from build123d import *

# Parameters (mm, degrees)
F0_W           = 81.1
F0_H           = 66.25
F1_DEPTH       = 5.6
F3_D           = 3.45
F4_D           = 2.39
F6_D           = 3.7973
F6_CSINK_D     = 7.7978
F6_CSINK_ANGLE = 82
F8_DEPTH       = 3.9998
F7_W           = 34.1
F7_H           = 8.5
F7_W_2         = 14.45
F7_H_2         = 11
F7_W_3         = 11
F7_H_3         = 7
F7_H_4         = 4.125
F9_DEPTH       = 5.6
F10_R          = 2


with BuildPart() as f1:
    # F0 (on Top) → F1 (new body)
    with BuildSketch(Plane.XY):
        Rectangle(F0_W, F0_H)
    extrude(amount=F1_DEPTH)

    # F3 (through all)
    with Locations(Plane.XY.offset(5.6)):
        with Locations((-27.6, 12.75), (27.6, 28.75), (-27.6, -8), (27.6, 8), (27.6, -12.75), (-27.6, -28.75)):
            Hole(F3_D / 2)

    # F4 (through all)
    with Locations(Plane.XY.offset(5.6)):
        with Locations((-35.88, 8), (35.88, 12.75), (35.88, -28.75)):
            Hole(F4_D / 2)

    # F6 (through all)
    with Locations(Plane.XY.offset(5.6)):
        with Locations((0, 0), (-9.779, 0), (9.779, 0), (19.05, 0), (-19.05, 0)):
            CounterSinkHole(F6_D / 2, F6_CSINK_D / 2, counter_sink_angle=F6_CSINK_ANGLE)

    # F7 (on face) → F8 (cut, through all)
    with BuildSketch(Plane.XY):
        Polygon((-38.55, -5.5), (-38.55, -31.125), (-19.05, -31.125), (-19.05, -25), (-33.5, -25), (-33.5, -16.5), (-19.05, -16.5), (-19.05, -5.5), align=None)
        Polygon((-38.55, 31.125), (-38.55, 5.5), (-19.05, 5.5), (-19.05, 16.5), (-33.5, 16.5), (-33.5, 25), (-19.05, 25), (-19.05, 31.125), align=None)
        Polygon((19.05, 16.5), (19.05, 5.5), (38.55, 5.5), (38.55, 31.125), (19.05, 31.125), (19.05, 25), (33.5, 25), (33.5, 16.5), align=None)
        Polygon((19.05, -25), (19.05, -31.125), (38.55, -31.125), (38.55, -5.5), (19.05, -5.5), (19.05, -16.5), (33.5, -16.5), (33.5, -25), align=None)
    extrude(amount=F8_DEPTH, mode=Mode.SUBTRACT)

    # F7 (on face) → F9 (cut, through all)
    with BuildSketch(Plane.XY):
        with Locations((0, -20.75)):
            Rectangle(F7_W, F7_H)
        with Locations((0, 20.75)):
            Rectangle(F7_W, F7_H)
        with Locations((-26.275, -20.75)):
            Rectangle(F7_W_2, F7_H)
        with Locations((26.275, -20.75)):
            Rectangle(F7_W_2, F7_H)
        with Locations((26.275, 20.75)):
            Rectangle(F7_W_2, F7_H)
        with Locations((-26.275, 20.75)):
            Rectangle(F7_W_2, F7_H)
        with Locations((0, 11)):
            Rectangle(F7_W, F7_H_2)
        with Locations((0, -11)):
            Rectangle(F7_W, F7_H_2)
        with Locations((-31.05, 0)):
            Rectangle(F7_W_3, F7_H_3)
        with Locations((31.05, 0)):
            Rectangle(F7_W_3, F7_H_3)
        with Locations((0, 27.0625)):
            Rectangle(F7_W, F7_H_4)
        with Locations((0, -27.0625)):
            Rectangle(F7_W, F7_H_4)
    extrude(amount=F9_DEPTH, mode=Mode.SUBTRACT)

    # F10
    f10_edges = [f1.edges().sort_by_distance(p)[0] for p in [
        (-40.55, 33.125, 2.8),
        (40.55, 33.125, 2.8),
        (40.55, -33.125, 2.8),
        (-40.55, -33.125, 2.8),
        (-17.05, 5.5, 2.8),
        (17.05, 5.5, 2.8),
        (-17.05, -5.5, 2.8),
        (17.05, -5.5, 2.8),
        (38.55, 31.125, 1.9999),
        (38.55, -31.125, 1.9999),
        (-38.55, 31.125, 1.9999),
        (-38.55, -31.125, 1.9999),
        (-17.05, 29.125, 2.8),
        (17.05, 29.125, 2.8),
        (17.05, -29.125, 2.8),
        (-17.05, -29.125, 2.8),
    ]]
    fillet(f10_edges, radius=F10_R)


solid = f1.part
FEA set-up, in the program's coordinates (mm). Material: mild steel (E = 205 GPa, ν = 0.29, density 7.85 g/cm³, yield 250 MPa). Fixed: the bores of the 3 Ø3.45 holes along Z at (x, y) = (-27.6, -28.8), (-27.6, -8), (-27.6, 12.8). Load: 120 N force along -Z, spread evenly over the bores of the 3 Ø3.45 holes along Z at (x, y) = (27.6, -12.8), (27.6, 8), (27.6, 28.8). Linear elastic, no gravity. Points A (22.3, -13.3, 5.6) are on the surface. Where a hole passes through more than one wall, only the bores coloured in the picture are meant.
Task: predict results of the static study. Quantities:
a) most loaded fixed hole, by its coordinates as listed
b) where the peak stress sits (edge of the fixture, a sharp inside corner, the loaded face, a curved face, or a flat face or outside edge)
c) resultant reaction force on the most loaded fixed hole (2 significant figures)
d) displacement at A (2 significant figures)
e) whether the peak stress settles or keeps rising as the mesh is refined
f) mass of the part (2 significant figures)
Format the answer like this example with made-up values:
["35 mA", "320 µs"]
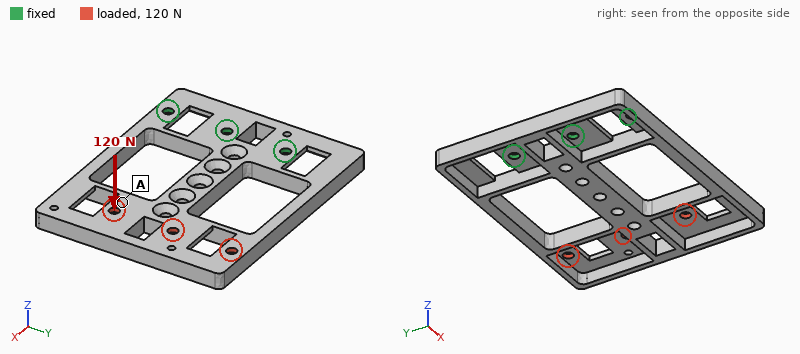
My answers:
["(-27.6, -8)", "edge of the fixture", "200 N", "0.24 mm", "keeps rising", "85 g"]
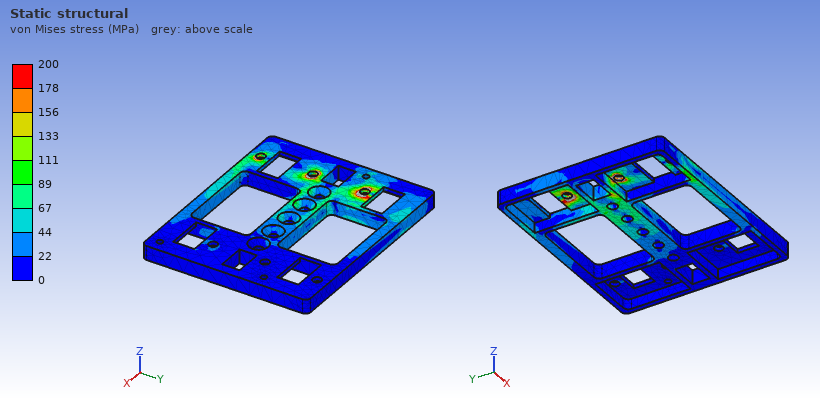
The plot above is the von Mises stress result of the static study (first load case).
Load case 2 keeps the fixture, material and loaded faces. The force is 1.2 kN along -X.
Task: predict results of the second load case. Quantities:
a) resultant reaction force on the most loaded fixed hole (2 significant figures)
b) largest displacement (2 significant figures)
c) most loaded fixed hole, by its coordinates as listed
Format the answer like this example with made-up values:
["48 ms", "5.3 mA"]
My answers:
["880 N", "0.11 mm", "(-27.6, 12.8)"]
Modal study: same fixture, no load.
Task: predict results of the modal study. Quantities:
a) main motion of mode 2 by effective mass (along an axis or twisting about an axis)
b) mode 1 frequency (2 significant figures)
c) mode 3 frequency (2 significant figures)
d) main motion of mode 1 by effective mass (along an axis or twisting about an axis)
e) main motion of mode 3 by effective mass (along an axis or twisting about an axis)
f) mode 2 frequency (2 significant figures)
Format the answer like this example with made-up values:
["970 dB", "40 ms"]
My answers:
["twisting about X", "510 Hz", "2400 Hz", "along Z", "along Y", "1100 Hz"]
